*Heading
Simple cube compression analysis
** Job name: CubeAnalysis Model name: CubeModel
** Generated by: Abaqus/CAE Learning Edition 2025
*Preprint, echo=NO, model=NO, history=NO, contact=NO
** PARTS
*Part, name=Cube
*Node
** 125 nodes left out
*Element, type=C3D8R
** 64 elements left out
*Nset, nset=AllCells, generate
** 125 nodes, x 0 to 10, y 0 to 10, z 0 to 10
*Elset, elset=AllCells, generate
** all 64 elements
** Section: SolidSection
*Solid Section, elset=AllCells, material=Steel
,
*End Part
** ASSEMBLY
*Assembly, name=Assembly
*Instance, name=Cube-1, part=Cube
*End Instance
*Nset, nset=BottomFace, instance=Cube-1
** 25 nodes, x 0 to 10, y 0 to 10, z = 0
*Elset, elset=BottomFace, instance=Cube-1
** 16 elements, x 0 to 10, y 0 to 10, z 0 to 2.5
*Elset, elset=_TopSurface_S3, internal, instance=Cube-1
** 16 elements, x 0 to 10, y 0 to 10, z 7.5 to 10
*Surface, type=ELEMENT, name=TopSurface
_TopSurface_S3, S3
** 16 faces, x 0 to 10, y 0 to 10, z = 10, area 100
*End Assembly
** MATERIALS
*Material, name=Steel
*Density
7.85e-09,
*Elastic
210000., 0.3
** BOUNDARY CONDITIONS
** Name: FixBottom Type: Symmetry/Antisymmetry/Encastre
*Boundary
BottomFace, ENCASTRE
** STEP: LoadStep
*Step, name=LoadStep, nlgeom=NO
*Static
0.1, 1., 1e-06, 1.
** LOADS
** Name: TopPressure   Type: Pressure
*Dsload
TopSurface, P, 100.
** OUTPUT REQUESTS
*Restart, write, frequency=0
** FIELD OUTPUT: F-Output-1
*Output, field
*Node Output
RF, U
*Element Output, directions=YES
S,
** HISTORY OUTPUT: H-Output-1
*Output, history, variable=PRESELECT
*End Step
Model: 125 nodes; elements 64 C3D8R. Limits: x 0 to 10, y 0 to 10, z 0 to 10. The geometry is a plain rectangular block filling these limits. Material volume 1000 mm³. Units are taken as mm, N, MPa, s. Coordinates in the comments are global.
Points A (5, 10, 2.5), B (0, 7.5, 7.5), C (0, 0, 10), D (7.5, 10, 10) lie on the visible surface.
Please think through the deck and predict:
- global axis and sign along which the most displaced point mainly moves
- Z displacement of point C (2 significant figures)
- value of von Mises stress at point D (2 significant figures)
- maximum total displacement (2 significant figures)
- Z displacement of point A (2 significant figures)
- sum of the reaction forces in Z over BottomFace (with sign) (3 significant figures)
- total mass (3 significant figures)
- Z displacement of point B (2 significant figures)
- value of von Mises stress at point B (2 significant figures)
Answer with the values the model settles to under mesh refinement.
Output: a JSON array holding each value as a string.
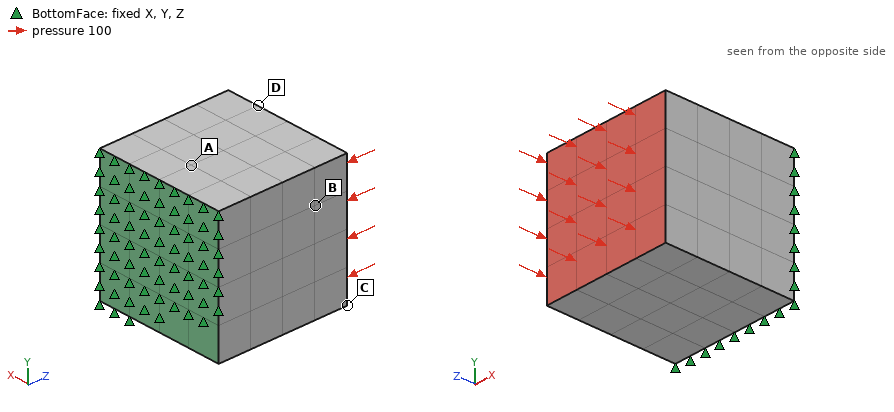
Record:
["-Z", "-0.0047 mm", "100 MPa", "0.0048 mm", "-0.0011 mm", "10000 N", "0.00785 kg", "-0.0034 mm", "99 MPa"]
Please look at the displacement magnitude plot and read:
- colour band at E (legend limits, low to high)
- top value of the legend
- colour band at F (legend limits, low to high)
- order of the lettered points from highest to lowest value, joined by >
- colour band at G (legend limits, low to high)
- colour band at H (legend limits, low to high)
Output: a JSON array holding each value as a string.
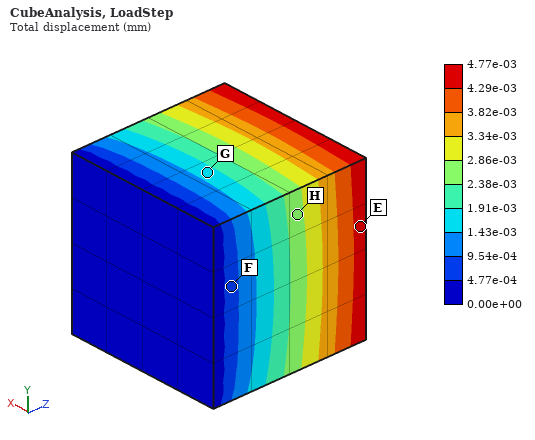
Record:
["4.29e-03 to 4.77e-03 mm", "4.77e-03 mm", "4.77e-04 to 9.54e-04 mm", "E > H > G > F", "1.43e-03 to 1.91e-03 mm", "2.38e-03 to 2.86e-03 mm"]
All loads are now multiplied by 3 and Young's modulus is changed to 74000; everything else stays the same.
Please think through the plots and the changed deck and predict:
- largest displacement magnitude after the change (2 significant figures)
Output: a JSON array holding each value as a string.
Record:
["0.041 mm"]
